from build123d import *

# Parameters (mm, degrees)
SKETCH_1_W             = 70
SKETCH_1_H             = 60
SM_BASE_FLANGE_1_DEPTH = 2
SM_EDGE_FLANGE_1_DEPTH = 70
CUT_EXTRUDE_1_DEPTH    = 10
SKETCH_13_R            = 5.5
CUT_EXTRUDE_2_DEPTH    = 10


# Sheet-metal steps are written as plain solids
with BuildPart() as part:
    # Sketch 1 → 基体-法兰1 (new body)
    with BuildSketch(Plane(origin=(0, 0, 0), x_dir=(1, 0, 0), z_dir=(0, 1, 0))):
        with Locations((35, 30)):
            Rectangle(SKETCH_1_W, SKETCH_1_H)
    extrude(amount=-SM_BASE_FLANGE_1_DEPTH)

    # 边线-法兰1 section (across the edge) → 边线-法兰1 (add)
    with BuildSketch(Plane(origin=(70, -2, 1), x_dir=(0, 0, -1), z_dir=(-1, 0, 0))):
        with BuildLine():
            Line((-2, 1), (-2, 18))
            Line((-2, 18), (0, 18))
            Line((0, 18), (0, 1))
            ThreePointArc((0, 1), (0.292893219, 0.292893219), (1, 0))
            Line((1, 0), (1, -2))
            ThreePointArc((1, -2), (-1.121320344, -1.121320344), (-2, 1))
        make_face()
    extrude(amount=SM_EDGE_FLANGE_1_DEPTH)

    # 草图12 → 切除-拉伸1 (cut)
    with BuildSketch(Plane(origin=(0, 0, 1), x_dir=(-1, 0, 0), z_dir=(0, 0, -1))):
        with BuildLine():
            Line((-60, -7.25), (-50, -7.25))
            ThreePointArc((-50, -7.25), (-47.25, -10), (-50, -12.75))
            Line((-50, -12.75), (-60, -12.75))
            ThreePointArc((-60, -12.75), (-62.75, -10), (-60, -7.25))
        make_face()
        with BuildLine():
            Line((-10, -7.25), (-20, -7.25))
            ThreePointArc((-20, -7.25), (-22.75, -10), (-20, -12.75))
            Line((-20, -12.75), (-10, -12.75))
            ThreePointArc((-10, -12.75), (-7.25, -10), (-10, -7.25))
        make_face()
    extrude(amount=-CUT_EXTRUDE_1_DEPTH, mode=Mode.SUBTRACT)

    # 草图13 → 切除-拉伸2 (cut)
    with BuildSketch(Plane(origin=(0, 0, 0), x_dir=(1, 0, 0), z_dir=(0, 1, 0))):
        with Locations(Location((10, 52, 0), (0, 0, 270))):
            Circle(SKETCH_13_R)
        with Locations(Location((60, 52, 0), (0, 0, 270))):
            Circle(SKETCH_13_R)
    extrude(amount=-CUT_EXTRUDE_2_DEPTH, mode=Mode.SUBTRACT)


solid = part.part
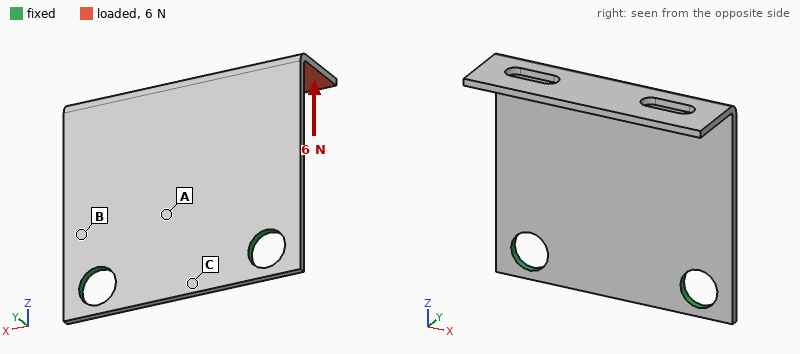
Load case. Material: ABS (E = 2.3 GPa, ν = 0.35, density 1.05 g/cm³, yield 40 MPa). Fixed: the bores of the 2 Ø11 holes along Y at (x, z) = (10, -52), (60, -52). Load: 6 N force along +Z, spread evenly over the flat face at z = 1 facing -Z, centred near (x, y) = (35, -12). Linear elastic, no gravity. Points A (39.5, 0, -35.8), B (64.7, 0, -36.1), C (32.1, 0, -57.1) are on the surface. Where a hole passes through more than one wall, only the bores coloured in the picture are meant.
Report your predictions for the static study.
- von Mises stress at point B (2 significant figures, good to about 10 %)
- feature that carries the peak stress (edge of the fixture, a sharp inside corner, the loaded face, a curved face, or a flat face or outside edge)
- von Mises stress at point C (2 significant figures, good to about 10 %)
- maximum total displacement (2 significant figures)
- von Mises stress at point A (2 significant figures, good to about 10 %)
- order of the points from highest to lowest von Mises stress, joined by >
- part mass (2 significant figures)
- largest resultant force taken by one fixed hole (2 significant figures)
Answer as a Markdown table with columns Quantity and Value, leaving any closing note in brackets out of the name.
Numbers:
| Quantity | Value |
|---|---|
| von Mises stress at point B | 1.4 MPa |
| feature that carries the peak stress | a flat face or outside edge |
| von Mises stress at point C | 0.30 MPa |
| maximum total displacement | 0.98 mm |
| von Mises stress at point A | 1.1 MPa |
| order of the points from highest to lowest von Mises stress, joined by > | B > A > C |
| part mass | 11 g |
| largest resultant force taken by one fixed hole | 3.1 N |
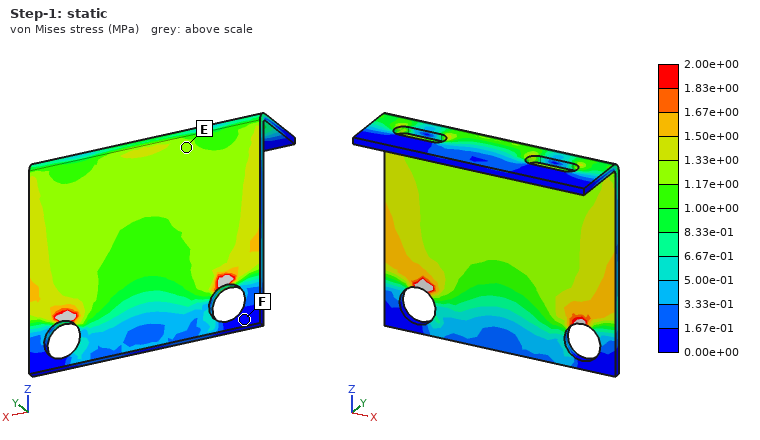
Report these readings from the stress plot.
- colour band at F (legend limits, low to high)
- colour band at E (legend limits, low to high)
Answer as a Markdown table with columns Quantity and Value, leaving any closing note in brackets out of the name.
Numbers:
| Quantity | Value |
|---|---|
| colour band at F | 0.00e+00 to 1.67e-01 MPa |
| colour band at E | 1.17e+00 to 1.33e+00 MPa |
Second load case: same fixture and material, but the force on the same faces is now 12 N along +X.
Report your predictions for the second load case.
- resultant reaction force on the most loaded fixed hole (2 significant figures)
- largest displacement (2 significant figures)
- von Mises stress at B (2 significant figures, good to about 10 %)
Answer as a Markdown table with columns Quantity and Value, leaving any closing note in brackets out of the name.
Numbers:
| Quantity | Value |
|---|---|
| resultant reaction force on the most loaded fixed hole | 13 N |
| largest displacement | 0.95 mm |
| von Mises stress at B | 1.9 MPa |
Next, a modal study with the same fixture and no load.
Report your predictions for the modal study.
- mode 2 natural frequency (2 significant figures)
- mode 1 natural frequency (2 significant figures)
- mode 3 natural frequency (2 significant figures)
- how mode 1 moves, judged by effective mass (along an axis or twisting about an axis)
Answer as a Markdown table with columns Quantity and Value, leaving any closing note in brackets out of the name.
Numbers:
| Quantity | Value |
|---|---|
| mode 2 natural frequency | 260 Hz |
| mode 1 natural frequency | 120 Hz |
| mode 3 natural frequency | 600 Hz |
| how mode 1 moves, judged by effective mass | along Y |
